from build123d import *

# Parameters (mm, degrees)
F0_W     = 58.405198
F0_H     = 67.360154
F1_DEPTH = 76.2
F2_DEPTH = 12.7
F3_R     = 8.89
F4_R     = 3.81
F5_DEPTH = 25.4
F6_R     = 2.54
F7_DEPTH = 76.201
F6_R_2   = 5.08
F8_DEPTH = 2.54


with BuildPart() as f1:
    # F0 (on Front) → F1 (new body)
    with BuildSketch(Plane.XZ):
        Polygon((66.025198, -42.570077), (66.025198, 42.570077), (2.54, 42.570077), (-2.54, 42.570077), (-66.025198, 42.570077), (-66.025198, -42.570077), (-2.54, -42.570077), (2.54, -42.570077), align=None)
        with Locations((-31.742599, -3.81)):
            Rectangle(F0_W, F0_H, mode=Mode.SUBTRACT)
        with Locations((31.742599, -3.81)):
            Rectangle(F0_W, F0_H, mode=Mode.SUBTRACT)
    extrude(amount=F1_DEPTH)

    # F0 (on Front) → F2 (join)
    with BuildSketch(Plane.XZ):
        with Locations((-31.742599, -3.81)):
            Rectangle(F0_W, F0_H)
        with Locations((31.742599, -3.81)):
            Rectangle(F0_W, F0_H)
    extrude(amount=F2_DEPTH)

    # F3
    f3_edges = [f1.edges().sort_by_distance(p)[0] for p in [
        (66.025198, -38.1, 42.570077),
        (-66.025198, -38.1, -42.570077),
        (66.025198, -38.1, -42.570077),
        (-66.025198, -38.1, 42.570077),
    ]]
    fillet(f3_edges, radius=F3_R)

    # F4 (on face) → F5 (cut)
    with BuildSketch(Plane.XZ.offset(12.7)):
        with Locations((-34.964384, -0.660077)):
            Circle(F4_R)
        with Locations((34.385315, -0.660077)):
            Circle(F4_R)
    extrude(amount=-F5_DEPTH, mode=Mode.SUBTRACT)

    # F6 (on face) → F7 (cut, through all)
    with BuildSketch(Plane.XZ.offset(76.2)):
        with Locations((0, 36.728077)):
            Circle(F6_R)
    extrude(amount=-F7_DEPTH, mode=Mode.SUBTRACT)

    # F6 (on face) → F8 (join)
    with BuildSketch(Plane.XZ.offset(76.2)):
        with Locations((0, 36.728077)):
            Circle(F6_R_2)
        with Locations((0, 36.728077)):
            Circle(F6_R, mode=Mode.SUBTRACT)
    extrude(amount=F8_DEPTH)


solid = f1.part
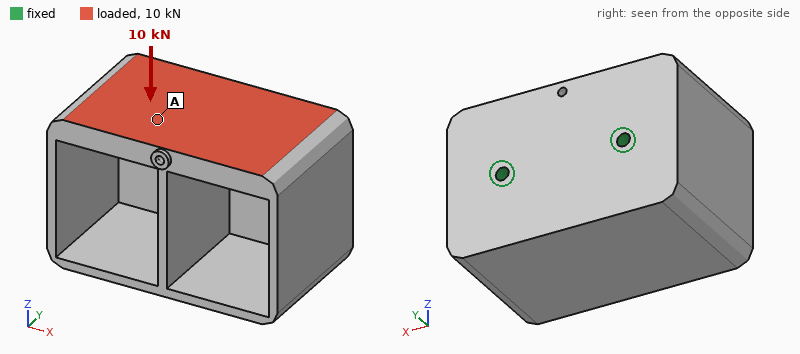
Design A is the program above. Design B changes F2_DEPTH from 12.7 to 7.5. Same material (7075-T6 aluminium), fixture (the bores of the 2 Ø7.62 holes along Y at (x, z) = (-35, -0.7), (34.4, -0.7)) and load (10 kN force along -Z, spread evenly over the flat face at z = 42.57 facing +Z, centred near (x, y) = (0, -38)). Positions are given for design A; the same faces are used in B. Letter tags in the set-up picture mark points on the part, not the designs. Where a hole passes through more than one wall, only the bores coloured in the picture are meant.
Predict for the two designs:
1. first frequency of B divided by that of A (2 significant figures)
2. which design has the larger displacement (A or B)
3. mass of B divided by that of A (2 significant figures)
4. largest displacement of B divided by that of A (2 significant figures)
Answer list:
0.53
B
0.88
3.5
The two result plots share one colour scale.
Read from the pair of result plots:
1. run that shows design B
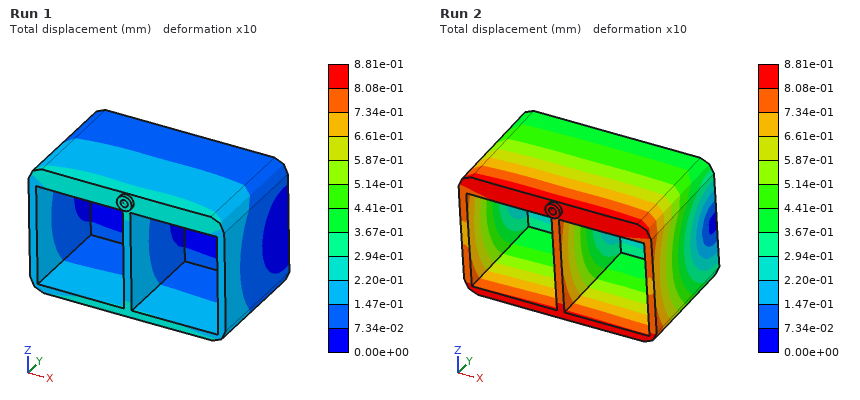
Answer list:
Run 2
